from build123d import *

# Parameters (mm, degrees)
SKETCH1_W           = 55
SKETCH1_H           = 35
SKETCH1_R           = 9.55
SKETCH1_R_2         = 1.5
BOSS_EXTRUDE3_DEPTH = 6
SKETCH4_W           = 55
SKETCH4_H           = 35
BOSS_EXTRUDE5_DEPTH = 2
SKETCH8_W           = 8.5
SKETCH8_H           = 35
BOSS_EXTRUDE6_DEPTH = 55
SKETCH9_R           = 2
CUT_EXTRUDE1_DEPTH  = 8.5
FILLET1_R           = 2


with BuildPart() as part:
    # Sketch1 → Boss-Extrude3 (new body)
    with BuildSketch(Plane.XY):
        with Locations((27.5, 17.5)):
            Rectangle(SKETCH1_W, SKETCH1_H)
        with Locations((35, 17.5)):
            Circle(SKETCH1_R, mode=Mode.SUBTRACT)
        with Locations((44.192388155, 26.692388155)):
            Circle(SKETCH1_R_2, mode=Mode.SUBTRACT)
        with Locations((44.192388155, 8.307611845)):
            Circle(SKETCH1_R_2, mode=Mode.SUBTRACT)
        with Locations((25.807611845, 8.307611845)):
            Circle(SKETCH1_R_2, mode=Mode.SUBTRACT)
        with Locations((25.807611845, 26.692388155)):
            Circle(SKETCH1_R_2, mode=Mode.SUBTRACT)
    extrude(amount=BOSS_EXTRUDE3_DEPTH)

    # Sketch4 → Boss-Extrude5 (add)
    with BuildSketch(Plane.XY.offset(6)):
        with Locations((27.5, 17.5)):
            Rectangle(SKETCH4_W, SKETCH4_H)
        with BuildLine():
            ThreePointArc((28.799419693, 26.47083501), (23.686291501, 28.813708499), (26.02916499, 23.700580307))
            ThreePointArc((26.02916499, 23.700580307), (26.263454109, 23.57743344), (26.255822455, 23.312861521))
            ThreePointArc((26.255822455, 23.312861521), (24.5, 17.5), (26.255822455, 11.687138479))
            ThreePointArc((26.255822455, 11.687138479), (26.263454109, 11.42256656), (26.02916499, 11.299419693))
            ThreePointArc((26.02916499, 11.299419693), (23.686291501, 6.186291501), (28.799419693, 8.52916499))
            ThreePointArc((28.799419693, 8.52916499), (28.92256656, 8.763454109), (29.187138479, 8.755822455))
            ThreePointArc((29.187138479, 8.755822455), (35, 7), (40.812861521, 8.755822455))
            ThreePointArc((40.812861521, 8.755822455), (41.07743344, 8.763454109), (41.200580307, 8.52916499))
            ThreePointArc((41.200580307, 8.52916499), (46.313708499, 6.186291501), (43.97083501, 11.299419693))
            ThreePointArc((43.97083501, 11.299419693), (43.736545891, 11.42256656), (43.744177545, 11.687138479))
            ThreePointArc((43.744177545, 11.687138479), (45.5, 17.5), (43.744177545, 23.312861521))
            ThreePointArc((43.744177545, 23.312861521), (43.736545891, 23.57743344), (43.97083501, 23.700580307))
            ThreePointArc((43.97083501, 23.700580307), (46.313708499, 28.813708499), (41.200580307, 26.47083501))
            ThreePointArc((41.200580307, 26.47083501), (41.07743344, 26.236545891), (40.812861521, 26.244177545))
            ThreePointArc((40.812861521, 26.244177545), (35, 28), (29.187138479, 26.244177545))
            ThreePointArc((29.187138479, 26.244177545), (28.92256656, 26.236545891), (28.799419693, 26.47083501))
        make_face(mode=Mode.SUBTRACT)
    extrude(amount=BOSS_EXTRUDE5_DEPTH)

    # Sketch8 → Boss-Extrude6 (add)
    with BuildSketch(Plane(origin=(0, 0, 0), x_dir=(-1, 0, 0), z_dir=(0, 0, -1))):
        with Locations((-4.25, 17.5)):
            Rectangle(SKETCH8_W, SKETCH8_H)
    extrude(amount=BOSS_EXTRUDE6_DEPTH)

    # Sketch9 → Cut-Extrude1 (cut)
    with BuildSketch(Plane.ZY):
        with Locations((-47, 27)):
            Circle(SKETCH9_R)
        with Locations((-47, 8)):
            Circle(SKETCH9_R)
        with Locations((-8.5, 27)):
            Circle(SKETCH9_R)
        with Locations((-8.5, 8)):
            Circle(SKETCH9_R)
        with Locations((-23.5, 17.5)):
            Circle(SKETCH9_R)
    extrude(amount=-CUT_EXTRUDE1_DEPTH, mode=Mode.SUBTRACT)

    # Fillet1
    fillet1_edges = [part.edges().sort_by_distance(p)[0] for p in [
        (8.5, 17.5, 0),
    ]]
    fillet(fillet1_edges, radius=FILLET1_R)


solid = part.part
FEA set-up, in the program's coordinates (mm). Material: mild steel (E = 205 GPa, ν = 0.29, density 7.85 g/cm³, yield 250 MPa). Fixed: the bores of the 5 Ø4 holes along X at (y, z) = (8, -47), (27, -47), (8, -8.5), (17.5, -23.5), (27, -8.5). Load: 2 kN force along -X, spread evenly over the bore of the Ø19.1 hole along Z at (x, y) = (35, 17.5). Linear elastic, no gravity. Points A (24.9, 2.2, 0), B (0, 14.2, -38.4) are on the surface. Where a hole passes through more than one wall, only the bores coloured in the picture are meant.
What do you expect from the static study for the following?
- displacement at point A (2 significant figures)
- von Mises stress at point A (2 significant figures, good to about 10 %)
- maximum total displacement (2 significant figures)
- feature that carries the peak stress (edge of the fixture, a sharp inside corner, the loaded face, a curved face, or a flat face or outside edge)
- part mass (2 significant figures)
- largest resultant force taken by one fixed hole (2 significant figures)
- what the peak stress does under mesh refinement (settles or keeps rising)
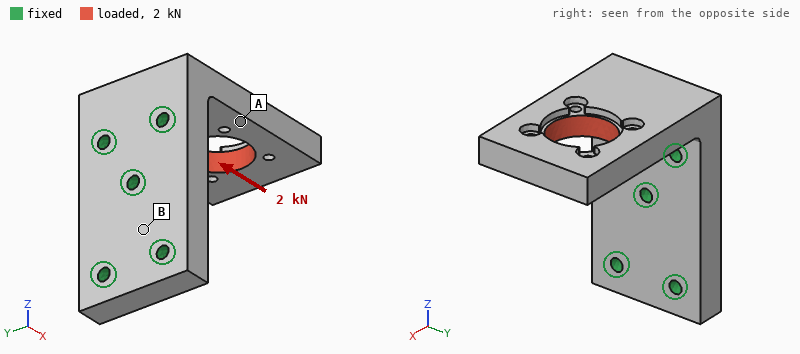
8.7 µm
16 MPa
16 µm
edge of the fixture
220 g
1.1 kN
keeps rising
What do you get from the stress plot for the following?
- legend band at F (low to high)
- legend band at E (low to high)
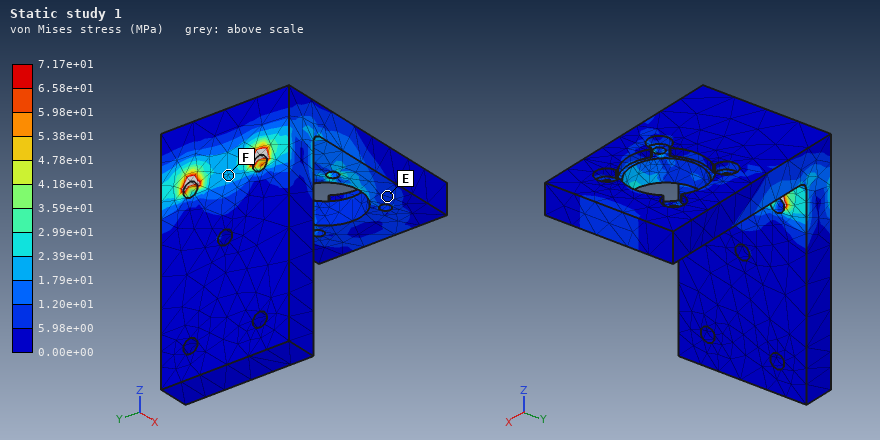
1.79e+01 to 2.39e+01 MPa
5.98e+00 to 1.20e+01 MPa
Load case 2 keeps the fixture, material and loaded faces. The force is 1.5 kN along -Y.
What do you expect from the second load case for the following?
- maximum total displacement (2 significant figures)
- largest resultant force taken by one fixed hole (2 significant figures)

37 µm
2.1 kN
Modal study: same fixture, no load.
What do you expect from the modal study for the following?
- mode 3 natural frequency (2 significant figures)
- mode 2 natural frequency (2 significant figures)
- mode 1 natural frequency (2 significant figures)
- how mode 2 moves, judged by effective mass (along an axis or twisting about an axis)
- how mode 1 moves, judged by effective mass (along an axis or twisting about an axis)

6100 Hz
4500 Hz
2100 Hz
along Y
along Z
